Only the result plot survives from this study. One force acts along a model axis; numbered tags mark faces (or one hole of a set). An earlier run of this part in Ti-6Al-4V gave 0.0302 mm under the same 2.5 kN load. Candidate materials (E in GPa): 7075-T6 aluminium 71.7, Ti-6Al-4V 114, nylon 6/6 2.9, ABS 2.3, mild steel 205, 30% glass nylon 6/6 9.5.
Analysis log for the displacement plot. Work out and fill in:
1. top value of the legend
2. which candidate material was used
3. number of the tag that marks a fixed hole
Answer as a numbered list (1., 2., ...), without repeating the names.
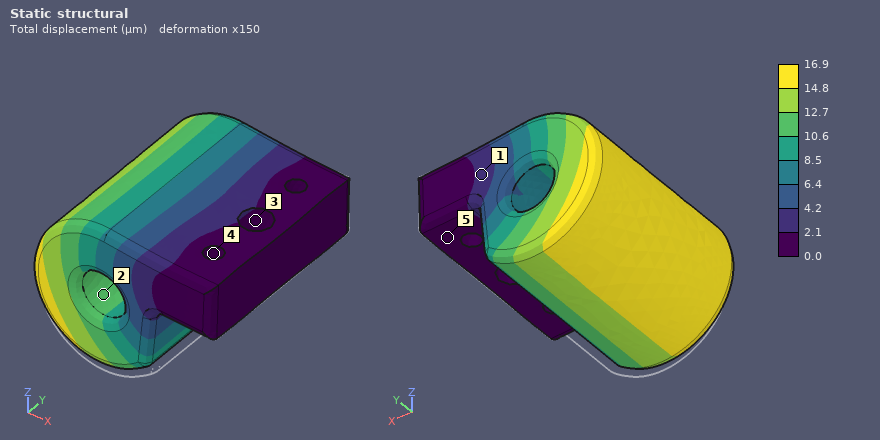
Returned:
1. 16.9 µm
2. mild steel
3. 4
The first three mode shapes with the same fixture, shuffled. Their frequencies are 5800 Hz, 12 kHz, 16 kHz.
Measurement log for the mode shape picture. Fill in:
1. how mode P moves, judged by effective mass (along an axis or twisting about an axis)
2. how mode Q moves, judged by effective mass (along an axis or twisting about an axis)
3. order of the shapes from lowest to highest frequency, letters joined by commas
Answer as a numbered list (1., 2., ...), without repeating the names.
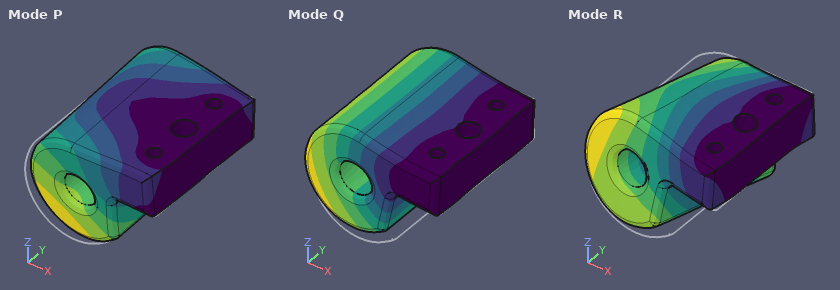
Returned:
1. along Y
2. along Z
3. Q, P, R
